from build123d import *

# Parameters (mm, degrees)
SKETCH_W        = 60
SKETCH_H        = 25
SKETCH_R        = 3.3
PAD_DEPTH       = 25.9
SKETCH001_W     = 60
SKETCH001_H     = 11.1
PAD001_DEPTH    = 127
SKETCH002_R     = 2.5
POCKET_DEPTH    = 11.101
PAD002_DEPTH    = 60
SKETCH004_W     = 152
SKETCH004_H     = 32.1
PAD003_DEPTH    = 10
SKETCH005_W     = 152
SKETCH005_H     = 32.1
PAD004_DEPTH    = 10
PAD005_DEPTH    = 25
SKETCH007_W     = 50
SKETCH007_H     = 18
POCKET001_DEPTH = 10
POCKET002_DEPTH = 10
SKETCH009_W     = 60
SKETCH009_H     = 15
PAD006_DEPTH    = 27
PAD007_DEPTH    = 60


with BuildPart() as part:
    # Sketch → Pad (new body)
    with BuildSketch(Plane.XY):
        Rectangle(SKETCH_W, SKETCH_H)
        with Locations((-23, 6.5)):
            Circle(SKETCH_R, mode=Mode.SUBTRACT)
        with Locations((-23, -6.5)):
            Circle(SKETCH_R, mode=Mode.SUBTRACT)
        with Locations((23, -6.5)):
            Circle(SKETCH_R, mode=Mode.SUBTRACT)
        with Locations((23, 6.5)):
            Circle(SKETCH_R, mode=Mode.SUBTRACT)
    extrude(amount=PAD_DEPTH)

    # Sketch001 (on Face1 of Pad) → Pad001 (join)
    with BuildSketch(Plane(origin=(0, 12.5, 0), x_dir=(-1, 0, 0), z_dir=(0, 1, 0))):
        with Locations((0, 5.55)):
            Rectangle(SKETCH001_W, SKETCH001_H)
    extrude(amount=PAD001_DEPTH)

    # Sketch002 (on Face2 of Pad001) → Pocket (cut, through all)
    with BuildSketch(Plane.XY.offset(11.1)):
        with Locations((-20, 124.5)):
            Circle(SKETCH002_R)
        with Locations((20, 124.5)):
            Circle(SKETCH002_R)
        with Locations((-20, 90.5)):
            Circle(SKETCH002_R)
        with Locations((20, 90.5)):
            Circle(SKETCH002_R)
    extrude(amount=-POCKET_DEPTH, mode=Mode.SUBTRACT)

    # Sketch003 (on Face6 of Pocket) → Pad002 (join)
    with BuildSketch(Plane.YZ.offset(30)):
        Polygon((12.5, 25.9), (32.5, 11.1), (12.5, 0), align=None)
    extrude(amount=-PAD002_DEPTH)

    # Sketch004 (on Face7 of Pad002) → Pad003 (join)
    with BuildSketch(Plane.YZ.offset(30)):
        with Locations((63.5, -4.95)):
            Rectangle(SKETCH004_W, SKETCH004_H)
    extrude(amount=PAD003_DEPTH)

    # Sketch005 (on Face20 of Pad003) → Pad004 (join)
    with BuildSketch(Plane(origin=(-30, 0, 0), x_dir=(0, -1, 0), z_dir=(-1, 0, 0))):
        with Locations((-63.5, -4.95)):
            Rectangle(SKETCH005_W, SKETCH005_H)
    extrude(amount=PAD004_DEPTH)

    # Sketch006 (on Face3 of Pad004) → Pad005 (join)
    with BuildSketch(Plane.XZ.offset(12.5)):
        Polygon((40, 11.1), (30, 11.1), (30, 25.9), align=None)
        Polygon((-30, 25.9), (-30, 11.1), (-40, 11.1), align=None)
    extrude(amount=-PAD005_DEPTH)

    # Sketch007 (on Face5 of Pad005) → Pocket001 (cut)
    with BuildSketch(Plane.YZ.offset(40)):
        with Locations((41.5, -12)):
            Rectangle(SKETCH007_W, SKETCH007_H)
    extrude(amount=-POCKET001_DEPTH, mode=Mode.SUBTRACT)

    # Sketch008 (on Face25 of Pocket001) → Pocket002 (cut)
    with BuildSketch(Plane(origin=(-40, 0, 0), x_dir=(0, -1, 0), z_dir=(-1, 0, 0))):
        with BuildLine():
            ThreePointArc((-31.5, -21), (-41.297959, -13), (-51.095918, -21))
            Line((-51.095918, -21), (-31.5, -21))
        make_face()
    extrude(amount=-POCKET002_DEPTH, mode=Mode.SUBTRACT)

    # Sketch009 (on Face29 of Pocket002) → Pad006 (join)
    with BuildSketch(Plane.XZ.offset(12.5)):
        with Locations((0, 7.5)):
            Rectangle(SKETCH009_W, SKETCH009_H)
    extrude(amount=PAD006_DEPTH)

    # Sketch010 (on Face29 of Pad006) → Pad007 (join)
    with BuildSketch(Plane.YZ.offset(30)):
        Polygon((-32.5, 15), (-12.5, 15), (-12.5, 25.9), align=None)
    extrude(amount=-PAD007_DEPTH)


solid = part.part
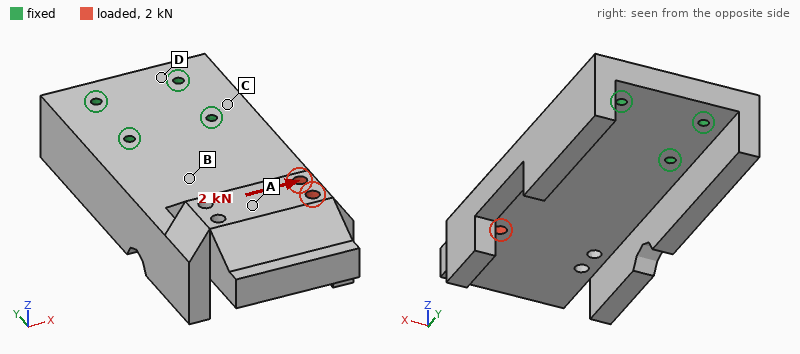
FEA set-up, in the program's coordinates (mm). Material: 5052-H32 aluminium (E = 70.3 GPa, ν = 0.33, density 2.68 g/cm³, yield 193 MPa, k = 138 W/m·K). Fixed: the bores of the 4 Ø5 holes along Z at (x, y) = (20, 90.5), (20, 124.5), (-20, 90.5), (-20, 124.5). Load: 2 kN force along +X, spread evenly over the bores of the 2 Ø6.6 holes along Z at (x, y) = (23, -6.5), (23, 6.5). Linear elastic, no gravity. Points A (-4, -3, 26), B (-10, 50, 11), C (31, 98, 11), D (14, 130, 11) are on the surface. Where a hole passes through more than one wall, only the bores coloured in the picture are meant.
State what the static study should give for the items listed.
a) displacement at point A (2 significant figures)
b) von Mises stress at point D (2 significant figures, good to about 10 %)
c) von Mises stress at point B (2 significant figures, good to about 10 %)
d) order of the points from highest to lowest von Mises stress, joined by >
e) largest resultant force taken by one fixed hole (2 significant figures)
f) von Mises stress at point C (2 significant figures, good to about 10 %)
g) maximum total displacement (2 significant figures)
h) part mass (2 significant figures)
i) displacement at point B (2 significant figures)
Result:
32 µm
3.6 MPa
7.7 MPa
B > C > D > A
2.9 kN
5.4 MPa
45 µm
670 g
11 µm
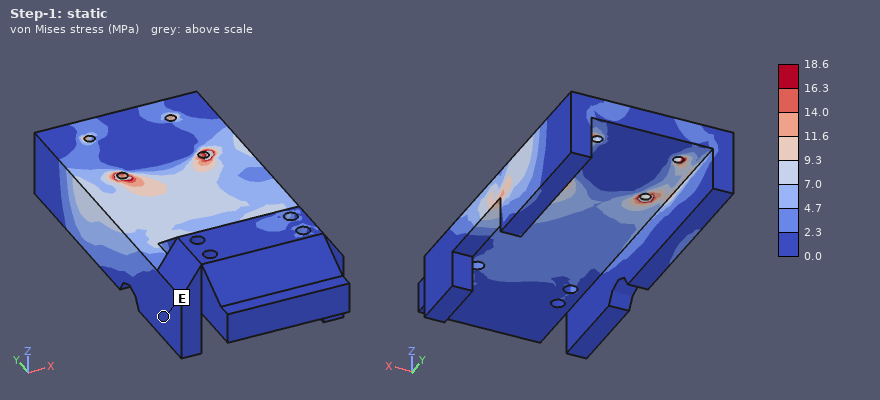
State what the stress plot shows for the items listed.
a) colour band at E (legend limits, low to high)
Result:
0.0 to 2.3 MPa
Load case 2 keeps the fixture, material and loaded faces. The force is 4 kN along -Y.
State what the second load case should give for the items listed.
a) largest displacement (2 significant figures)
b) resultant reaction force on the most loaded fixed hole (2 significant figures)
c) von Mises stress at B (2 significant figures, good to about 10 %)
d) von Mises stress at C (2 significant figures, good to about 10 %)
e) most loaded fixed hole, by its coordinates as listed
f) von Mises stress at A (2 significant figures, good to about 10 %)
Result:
0.11 mm
2.9 kN
9.8 MPa
7.1 MPa
(20, 90.5)
3.5 MPa
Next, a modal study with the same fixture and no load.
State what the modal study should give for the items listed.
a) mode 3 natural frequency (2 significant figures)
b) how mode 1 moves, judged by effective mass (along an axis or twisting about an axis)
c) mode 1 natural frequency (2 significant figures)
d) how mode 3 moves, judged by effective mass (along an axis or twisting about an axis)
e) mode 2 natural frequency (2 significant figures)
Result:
2300 Hz
along Z
730 Hz
along X
2000 Hz
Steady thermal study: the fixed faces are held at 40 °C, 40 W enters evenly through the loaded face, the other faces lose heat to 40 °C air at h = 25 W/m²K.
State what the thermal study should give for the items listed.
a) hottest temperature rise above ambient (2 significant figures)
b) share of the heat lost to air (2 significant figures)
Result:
22 K
27 %
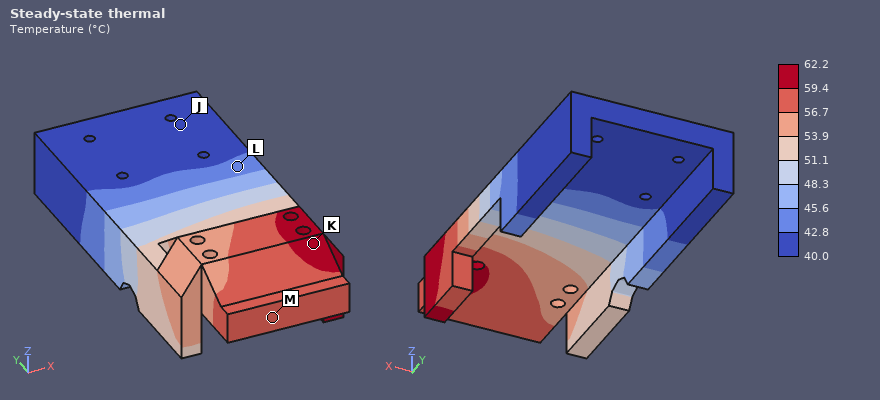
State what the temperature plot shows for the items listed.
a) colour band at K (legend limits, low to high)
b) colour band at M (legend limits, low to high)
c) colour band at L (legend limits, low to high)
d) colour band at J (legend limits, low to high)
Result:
59.4 to 62.2 °C
56.7 to 59.4 °C
42.8 to 45.6 °C
40.0 to 42.8 °C
